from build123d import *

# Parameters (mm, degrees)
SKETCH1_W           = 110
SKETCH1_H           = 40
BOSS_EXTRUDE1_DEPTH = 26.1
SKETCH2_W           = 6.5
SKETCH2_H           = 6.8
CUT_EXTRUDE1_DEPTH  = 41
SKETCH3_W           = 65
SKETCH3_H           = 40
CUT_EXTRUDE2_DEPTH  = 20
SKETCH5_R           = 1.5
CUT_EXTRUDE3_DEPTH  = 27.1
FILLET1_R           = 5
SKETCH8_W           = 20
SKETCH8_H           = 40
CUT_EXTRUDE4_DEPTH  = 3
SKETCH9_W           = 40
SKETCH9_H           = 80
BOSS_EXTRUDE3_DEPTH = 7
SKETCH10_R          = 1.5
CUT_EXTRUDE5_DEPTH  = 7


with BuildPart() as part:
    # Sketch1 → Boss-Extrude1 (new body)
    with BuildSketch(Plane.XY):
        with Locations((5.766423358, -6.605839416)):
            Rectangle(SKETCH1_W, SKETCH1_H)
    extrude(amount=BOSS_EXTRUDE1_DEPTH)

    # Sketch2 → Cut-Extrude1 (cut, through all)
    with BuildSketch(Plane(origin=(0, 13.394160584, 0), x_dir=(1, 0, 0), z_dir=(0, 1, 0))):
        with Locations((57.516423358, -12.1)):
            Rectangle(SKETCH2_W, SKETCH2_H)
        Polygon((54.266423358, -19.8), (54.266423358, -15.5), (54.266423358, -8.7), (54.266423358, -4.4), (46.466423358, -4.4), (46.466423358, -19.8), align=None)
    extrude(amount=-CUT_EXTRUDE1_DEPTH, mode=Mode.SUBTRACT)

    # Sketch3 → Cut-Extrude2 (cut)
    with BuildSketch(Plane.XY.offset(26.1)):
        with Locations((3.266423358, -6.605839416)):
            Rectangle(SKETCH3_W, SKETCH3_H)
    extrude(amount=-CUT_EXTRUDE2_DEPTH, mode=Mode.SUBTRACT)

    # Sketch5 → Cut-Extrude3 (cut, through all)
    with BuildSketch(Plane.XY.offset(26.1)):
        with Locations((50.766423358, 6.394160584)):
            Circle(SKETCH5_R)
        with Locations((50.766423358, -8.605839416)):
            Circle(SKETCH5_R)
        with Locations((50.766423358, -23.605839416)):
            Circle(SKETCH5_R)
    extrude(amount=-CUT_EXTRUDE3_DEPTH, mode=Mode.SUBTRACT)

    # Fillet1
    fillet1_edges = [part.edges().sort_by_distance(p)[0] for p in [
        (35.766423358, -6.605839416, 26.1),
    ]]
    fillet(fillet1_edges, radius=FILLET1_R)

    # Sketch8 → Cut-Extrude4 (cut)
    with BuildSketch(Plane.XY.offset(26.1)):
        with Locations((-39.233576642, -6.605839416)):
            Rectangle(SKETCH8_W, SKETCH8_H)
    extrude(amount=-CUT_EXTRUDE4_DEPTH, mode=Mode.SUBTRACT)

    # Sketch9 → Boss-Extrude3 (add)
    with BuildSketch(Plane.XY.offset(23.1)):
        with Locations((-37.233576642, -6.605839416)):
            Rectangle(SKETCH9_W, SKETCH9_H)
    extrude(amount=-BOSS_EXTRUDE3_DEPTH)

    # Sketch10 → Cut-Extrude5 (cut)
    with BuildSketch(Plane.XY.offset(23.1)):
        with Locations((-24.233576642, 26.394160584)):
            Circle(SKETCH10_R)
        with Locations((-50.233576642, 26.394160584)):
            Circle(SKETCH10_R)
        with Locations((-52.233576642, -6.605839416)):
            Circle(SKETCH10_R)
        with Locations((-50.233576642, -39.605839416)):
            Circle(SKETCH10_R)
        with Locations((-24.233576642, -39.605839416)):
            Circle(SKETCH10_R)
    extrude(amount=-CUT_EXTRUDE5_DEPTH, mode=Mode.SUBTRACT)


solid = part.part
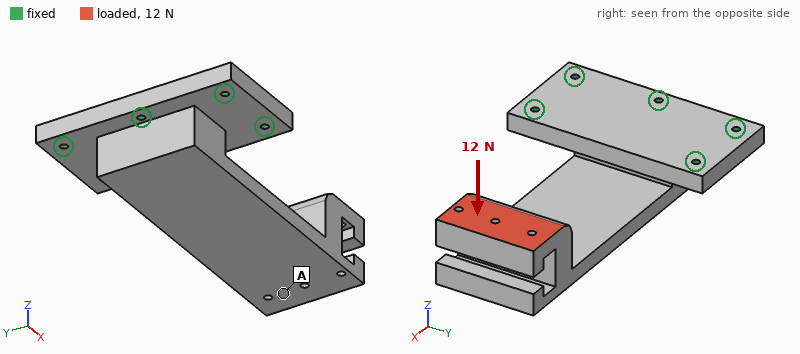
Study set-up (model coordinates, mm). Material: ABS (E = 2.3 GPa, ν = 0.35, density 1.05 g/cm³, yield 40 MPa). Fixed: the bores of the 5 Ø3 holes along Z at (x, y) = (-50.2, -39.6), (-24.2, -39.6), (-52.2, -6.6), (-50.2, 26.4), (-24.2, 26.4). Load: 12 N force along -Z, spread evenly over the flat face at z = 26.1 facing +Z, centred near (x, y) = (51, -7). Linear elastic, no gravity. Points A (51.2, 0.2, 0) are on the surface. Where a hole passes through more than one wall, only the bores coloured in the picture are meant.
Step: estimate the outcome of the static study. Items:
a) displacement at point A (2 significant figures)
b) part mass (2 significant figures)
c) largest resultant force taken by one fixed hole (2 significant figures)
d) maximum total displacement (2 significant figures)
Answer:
1.4 mm
73 g
21 N
1.7 mm
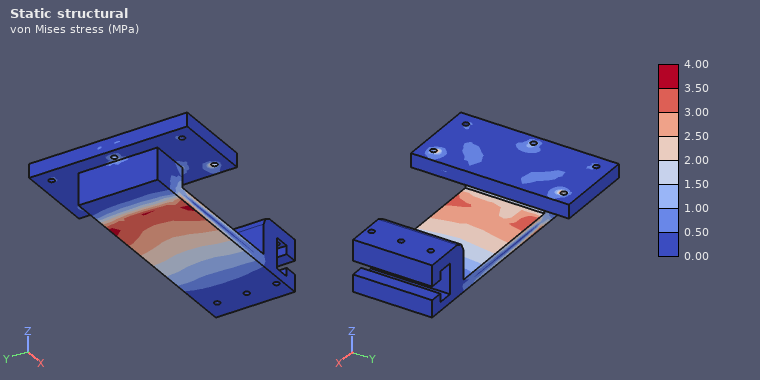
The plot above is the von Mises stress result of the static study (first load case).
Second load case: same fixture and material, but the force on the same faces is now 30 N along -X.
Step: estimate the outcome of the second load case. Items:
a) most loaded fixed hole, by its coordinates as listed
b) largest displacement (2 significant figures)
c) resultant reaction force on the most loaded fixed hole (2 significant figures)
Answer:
(-52.2, -6.6)
1.7 mm
16 N
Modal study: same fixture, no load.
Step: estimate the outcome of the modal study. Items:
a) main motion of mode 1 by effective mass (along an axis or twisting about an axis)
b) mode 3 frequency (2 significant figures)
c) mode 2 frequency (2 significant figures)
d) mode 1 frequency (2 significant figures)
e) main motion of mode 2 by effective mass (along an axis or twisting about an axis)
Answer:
along Z
610 Hz
340 Hz
100 Hz
along Y
